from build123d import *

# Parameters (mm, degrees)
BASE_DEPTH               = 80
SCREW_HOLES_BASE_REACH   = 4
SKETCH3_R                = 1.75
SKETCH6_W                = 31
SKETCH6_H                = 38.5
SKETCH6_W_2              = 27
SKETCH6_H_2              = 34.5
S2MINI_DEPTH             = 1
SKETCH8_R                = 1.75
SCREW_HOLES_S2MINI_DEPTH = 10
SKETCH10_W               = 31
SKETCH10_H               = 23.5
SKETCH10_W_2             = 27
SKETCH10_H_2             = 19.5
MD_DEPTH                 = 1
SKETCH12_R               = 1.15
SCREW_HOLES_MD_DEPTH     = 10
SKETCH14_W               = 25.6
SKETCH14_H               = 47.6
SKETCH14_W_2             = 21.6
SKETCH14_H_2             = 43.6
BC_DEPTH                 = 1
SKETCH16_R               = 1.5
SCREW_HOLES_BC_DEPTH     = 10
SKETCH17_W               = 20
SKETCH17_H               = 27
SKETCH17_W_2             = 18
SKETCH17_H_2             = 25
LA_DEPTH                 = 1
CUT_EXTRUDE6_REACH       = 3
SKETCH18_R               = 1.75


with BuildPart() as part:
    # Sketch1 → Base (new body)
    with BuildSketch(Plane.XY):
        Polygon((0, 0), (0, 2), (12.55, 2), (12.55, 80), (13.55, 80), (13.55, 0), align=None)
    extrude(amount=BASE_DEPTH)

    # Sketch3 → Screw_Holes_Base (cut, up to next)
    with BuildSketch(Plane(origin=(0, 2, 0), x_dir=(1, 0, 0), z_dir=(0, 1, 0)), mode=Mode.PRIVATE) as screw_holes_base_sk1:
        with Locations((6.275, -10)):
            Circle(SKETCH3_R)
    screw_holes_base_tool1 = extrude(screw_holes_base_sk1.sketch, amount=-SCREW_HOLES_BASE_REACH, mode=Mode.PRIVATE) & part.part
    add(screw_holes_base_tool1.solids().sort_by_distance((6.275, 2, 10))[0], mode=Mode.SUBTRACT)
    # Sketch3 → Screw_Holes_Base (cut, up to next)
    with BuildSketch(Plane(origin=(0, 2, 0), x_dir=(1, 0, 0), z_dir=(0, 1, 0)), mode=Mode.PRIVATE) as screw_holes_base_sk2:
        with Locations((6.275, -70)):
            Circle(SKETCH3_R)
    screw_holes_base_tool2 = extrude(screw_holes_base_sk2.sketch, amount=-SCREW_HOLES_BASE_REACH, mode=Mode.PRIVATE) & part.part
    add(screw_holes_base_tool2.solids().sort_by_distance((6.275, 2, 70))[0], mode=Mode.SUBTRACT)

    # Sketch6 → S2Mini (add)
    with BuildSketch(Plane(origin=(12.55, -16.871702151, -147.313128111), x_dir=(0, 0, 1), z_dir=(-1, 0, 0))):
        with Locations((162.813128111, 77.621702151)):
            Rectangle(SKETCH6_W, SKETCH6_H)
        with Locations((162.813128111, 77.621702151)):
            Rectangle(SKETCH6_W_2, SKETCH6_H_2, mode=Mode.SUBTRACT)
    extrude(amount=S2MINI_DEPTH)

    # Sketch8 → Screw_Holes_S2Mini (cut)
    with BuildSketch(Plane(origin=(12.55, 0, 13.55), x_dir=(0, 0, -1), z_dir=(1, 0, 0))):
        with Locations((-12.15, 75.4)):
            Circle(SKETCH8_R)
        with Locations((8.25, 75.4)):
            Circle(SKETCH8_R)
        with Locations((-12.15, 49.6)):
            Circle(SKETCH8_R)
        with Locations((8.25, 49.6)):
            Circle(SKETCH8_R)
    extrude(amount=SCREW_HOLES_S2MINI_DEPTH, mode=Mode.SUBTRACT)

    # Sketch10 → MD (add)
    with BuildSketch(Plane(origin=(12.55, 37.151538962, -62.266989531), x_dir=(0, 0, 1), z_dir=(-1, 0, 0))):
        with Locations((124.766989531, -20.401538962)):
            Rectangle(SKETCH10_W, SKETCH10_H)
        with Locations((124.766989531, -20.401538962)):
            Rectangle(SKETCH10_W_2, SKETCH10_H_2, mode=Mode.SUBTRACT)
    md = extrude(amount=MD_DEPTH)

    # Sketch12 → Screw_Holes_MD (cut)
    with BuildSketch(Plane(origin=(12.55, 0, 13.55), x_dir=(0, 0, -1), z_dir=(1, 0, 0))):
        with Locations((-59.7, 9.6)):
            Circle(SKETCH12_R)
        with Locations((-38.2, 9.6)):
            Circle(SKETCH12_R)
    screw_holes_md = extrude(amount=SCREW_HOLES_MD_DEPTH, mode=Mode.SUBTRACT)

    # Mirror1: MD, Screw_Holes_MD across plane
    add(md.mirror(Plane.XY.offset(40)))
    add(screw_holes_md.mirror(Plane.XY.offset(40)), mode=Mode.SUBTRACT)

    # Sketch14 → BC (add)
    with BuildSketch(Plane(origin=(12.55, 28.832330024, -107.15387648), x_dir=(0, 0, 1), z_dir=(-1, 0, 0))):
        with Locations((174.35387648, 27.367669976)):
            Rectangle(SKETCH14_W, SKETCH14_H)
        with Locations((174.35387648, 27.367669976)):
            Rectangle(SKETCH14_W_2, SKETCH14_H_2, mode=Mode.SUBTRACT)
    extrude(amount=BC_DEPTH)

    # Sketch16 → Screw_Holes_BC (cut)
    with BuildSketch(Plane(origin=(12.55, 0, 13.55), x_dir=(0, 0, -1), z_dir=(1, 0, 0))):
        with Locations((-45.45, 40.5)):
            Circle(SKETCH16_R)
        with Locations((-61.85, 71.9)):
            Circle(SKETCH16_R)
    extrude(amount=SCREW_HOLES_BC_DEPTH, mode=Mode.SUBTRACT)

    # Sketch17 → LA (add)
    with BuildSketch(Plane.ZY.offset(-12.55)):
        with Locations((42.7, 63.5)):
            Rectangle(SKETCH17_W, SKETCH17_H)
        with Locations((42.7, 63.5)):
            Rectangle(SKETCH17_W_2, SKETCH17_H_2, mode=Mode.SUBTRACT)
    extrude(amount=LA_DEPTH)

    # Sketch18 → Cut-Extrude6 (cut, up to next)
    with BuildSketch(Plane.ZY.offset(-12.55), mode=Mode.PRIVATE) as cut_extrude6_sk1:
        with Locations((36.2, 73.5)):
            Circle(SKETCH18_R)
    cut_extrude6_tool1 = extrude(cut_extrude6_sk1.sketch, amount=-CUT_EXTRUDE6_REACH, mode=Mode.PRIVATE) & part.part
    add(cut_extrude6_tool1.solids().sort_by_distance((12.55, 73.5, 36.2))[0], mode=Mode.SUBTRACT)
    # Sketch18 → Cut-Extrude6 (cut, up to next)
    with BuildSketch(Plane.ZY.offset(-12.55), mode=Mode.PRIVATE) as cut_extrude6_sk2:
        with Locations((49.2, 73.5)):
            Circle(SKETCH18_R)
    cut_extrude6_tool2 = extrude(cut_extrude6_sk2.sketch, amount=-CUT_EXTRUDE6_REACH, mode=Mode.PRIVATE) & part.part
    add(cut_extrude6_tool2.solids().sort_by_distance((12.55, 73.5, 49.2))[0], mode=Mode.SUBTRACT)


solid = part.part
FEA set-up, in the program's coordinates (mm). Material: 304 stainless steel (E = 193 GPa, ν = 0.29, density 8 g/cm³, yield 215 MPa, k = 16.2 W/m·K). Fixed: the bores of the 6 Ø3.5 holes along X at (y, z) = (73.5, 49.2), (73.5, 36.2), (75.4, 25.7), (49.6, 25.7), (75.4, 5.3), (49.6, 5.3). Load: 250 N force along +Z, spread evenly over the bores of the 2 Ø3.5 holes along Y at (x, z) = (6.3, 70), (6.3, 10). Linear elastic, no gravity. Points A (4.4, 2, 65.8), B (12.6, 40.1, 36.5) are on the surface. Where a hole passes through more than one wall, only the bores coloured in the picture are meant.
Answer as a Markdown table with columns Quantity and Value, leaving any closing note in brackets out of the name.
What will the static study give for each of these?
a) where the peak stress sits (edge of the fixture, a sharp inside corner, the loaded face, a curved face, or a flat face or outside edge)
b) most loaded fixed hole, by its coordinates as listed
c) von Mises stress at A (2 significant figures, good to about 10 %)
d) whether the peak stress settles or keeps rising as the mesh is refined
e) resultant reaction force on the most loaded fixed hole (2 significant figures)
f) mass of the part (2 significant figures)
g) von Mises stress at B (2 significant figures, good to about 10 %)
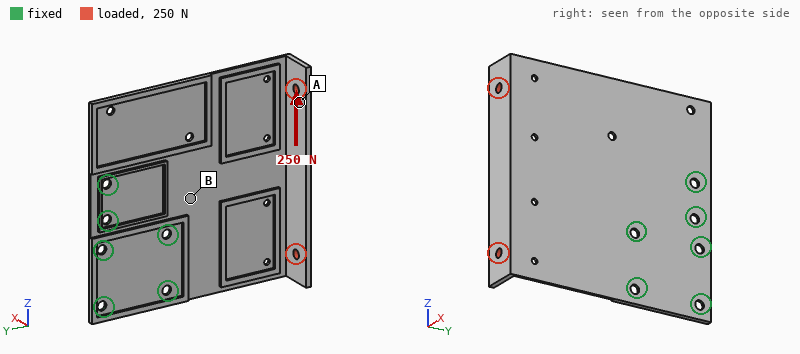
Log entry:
| Quantity | Value |
|---|---|
| where the peak stress sits | edge of the fixture |
| most loaded fixed hole, by its coordinates as listed | (49.6, 5.3) |
| von Mises stress at A | 19 MPa |
| whether the peak stress settles or keeps rising as the mesh is refined | keeps rising |
| resultant reaction force on the most loaded fixed hole | 280 N |
| mass of the part | 75 g |
| von Mises stress at B | 56 MPa |
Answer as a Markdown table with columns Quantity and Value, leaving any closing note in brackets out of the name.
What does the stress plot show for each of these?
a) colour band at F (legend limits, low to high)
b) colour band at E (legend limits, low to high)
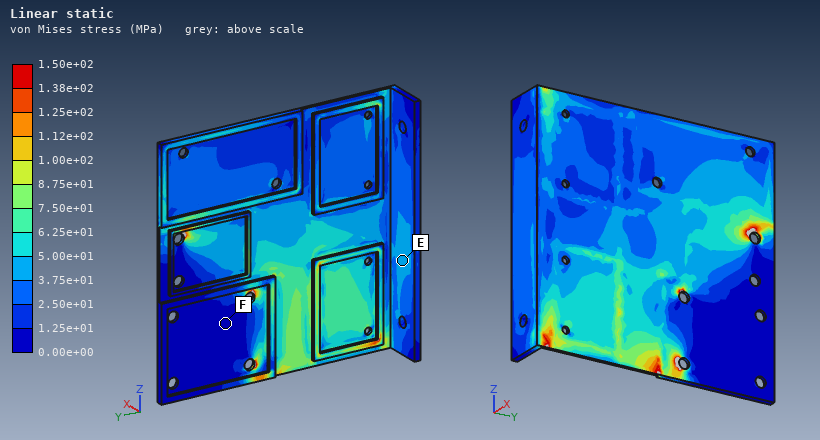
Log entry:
| Quantity | Value |
|---|---|
| colour band at F | 0.00e+00 to 1.25e+01 MPa |
| colour band at E | 3.75e+01 to 5.00e+01 MPa |
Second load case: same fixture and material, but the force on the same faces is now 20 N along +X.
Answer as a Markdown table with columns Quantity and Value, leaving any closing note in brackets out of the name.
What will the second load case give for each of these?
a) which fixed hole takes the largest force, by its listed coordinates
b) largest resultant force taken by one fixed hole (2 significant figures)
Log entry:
| Quantity | Value |
|---|---|
| which fixed hole takes the largest force, by its listed coordinates | (49.6, 25.7) |
| largest resultant force taken by one fixed hole | 58 N |
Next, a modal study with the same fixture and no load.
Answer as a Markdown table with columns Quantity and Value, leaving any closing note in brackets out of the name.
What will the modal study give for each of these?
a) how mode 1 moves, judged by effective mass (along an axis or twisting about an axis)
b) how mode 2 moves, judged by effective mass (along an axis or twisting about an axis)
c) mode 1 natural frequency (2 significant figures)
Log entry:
| Quantity | Value |
|---|---|
| how mode 1 moves, judged by effective mass | along X |
| how mode 2 moves, judged by effective mass | twisting about Y |
| mode 1 natural frequency | 180 Hz |
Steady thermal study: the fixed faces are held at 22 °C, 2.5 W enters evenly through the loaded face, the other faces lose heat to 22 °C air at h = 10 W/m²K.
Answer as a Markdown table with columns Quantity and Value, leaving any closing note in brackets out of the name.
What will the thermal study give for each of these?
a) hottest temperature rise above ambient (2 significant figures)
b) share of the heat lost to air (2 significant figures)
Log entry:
| Quantity | Value |
|---|---|
| hottest temperature rise above ambient | 53 K |
| share of the heat lost to air | 85 % |
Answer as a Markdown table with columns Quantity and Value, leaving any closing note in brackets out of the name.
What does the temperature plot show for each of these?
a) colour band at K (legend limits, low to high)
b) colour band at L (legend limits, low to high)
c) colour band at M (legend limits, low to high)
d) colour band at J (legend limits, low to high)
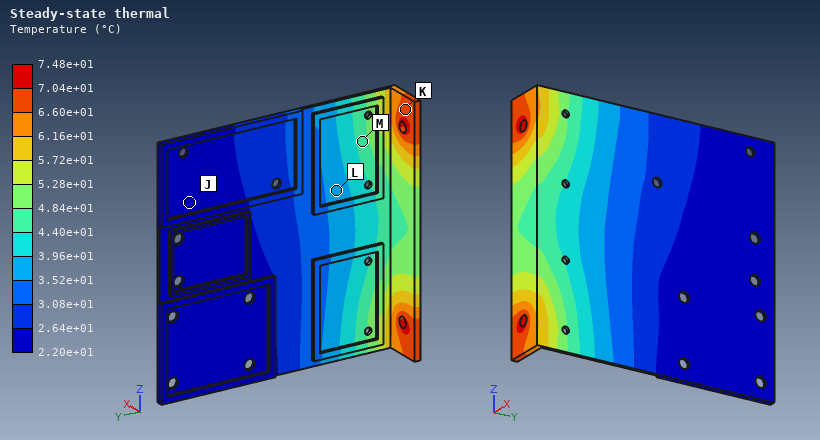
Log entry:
| Quantity | Value |
|---|---|
| colour band at K | 6.60e+01 to 7.04e+01 °C |
| colour band at L | 3.52e+01 to 3.96e+01 °C |
| colour band at M | 4.40e+01 to 4.84e+01 °C |
| colour band at J | 2.20e+01 to 2.64e+01 °C |
